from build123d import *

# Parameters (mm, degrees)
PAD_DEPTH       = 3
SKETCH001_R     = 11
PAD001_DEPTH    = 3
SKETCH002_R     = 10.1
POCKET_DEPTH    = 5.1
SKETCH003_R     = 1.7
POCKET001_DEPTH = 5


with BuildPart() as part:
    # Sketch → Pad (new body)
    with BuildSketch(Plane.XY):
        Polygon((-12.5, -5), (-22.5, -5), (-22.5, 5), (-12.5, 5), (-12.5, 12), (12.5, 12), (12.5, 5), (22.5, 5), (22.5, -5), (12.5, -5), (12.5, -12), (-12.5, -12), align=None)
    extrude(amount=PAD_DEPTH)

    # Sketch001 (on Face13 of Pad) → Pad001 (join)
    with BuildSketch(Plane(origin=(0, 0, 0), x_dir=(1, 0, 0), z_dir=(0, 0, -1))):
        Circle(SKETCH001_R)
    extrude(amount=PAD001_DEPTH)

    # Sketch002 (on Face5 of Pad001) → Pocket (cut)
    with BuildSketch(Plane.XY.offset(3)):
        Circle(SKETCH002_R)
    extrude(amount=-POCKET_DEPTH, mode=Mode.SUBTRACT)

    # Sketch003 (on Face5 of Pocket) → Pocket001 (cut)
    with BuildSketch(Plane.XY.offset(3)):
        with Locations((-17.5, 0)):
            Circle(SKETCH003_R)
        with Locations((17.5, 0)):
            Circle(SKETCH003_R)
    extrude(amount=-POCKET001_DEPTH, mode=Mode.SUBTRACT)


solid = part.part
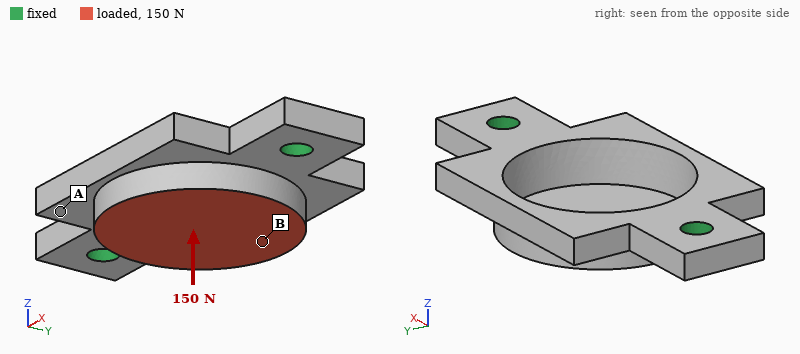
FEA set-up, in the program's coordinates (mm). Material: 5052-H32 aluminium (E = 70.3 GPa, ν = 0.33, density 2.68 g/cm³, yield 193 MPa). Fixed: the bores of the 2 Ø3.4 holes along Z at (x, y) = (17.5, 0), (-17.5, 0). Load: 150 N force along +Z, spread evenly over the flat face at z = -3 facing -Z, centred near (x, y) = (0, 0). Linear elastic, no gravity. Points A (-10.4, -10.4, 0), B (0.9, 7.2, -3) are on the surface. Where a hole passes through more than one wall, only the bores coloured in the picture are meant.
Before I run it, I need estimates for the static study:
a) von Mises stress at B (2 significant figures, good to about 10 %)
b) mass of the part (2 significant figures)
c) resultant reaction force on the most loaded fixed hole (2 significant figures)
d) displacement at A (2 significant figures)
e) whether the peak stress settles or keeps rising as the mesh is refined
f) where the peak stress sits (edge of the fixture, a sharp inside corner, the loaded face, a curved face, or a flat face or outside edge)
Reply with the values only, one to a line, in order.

19 MPa
5.0 g
110 N
5.1 µm
keeps rising
edge of the fixture
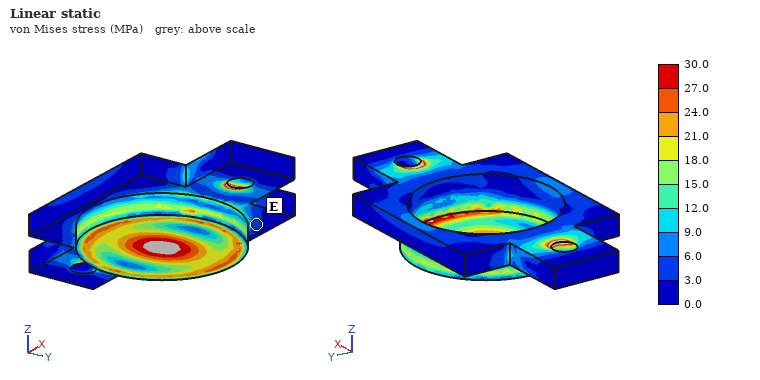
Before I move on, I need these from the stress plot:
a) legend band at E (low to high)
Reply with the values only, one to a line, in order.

3.0 to 6.0 MPa
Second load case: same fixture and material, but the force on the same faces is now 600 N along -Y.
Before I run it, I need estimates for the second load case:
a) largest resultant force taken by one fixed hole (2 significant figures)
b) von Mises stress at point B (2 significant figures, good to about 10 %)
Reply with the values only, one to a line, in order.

300 N
14 MPa
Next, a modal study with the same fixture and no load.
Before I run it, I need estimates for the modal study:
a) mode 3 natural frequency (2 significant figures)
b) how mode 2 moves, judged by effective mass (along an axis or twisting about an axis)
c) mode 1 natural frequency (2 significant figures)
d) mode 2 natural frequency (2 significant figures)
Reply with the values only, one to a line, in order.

19 kHz
along Z
8400 Hz
13 kHz
